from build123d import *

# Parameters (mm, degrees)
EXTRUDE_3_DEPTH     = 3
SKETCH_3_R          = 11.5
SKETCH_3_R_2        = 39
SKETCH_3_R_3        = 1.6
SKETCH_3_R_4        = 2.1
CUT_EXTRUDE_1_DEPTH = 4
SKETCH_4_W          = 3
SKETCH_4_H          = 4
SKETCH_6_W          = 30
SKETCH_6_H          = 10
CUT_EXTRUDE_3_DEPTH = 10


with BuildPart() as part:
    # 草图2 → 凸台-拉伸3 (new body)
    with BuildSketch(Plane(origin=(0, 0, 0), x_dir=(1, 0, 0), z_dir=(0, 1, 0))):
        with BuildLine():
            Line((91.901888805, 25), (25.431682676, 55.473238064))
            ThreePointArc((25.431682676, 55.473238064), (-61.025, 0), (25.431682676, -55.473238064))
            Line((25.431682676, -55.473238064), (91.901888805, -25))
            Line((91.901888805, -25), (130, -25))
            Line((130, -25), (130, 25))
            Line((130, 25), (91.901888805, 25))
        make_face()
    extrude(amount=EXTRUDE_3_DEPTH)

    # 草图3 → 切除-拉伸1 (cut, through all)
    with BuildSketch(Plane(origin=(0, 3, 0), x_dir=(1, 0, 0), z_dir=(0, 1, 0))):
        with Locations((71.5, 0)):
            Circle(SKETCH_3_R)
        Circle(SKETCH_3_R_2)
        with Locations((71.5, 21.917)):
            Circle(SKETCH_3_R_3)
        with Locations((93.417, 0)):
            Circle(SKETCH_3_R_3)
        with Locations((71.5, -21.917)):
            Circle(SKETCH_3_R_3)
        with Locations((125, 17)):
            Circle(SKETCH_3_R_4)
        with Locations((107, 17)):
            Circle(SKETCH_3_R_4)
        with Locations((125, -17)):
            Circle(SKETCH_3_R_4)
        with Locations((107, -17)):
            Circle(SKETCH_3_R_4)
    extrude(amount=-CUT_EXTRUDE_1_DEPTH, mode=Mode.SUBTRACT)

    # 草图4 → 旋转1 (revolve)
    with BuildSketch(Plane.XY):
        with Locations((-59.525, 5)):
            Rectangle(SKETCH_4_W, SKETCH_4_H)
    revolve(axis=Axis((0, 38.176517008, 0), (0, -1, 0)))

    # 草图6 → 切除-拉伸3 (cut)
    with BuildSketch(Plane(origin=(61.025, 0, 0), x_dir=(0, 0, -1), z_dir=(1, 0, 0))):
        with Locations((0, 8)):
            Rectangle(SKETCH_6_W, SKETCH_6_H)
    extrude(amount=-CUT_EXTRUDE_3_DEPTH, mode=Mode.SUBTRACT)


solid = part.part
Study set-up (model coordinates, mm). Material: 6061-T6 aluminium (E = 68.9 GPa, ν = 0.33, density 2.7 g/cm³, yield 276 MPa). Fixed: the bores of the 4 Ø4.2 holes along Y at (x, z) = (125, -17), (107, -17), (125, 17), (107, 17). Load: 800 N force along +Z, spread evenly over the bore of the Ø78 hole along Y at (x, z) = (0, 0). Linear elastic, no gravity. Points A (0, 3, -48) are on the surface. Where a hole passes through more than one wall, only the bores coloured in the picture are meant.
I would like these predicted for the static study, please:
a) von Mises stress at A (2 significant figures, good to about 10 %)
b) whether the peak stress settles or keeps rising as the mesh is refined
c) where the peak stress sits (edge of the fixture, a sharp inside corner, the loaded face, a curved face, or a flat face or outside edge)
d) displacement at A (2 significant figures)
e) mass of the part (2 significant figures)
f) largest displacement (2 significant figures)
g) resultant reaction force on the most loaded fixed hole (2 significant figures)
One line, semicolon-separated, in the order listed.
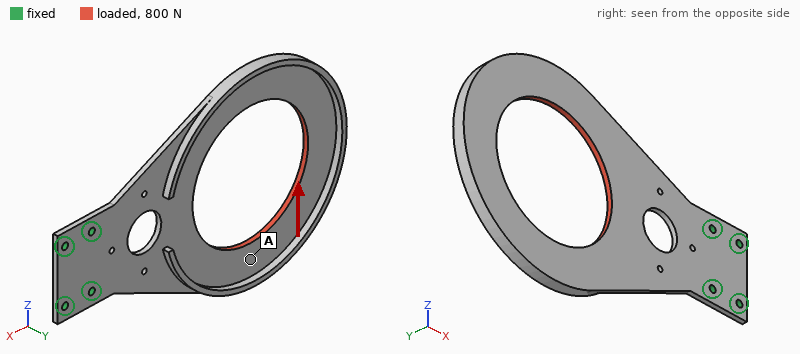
9.6 MPa; keeps rising; edge of the fixture; 0.27 mm; 99 g; 0.40 mm; 2.1 kN
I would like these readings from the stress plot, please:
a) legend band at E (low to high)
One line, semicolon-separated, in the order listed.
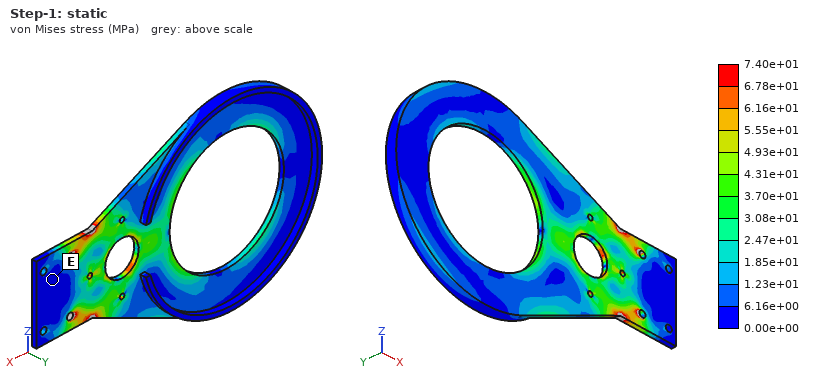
0.00e+00 to 6.16e+00 MPa
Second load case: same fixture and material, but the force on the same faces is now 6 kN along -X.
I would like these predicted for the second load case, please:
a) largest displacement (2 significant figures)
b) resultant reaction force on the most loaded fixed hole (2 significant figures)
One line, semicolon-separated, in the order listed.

0.20 mm; 2.4 kN
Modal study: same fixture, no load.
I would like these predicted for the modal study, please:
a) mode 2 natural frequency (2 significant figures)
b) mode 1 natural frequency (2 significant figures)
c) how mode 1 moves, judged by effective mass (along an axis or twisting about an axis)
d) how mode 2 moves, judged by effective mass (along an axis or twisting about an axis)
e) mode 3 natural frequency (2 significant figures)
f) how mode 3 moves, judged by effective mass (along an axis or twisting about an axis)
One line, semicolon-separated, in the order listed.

230 Hz; 75 Hz; along Y; twisting about X; 560 Hz; along Y
